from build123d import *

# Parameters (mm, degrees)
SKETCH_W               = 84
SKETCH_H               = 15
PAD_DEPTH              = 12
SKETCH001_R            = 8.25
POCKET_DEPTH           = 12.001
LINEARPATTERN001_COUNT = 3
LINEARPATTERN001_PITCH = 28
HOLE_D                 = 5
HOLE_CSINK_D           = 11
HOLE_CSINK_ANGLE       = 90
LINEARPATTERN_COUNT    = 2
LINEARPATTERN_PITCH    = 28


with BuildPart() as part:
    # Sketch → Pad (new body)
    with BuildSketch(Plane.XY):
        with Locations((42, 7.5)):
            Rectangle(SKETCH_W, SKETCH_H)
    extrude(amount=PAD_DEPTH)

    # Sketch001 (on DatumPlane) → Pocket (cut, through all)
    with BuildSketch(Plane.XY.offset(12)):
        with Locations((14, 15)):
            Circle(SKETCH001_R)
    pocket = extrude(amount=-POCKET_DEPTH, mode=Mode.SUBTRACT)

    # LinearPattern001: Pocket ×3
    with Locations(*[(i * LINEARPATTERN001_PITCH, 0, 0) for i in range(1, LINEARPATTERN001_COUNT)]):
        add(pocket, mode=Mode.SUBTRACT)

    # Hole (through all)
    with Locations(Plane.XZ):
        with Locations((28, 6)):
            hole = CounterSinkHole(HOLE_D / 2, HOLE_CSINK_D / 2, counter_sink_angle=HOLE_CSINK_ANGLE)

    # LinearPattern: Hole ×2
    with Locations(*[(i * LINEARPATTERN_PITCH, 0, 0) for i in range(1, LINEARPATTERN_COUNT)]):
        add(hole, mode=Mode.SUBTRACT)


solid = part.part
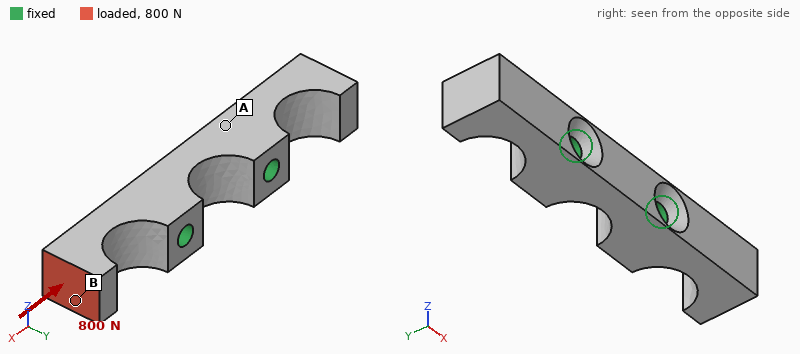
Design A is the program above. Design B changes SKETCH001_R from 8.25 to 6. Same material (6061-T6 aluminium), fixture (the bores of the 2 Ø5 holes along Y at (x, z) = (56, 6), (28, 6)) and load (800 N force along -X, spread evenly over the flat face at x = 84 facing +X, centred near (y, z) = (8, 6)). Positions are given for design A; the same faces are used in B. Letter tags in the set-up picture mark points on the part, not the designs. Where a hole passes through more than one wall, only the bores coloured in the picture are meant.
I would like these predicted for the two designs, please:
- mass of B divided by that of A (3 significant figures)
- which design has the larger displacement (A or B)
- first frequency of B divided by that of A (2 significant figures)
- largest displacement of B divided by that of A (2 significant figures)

1.17
A
1.2
0.30
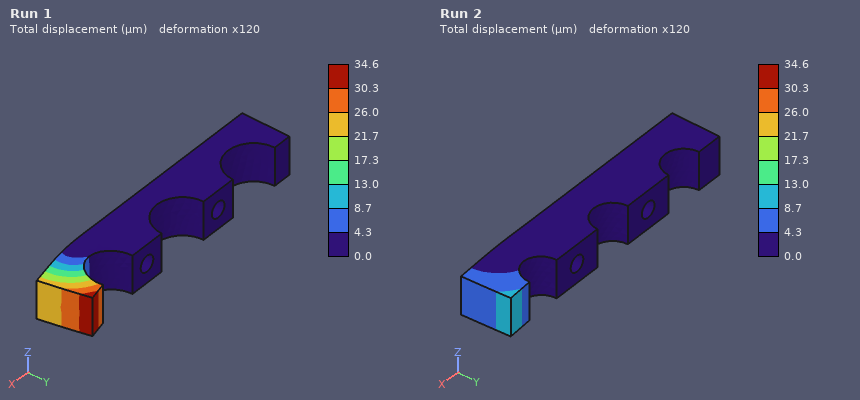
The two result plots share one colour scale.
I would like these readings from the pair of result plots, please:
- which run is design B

Run 2
